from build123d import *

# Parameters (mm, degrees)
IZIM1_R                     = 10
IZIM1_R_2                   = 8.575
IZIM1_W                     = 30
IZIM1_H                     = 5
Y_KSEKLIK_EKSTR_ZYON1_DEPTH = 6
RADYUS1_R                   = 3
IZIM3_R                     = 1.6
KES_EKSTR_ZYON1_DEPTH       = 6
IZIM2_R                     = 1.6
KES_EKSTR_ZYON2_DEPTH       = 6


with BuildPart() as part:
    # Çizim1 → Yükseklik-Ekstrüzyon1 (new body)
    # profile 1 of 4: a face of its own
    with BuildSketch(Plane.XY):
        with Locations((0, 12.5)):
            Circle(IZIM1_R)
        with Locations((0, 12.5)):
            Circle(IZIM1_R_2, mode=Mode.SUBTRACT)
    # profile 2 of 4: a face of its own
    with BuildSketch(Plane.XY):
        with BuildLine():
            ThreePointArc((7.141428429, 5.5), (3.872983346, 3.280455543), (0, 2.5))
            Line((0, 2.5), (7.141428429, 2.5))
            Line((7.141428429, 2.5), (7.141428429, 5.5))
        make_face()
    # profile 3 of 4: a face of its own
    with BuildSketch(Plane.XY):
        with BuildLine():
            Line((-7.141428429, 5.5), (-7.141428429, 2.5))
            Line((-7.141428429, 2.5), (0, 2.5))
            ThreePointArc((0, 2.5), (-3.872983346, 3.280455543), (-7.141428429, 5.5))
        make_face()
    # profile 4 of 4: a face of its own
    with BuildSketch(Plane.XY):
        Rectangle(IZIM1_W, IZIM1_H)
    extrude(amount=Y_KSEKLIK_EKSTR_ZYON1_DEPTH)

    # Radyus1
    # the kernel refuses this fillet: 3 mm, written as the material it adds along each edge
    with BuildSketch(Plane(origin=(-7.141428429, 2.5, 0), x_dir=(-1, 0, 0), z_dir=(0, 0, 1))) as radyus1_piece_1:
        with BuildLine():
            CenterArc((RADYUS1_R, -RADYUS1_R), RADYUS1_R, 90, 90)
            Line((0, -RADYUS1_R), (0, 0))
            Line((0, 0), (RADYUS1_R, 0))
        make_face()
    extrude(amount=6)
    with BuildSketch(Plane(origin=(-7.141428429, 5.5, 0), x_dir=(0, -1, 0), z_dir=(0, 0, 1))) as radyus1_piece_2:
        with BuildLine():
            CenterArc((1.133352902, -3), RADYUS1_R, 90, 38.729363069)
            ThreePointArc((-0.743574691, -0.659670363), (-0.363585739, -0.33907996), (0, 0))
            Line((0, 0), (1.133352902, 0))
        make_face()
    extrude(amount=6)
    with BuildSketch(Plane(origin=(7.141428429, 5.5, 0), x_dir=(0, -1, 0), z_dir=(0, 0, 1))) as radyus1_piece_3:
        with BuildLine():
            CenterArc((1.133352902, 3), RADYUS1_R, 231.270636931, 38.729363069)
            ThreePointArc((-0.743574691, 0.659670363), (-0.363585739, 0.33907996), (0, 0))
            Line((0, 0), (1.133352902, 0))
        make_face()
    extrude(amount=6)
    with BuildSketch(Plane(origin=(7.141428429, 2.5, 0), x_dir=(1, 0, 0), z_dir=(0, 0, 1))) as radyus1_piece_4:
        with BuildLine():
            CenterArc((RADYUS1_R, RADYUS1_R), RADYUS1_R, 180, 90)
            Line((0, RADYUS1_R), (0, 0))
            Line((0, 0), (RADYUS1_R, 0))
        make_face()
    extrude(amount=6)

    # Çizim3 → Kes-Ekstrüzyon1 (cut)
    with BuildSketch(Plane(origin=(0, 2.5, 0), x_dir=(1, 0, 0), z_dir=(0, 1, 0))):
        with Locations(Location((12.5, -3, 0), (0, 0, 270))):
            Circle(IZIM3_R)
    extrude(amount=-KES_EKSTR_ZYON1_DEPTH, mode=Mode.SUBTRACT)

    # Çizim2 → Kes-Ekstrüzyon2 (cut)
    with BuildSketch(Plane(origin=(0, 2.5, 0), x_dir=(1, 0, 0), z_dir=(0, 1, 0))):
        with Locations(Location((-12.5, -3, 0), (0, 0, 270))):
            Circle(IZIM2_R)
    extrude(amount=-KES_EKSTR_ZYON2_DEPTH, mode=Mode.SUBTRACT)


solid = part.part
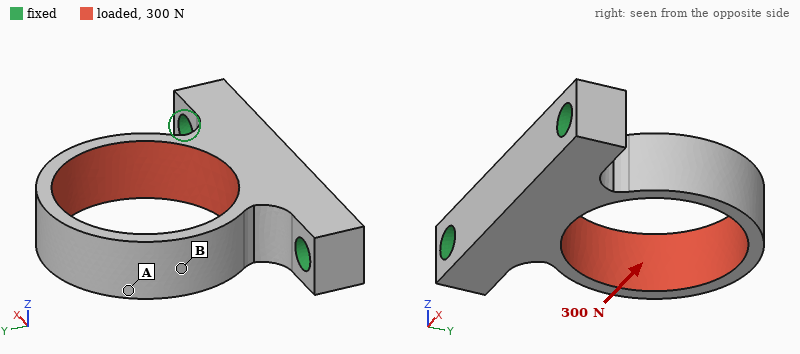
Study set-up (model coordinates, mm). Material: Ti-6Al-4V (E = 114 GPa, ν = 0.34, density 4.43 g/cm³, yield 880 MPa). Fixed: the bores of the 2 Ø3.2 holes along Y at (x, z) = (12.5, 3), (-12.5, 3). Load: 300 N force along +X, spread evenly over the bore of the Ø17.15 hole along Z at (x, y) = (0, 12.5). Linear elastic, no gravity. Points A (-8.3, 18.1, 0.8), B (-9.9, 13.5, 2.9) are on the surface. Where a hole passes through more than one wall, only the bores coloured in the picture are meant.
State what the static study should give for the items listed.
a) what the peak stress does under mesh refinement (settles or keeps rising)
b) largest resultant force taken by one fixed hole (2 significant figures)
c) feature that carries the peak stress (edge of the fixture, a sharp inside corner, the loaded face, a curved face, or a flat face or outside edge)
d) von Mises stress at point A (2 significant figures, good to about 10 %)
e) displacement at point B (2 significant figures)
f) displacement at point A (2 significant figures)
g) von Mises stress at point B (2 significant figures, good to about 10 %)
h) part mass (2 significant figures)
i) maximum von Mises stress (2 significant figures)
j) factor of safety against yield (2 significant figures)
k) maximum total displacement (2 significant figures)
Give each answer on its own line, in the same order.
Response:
settles
240 N
the loaded face
130 MPa
0.11 mm
0.15 mm
46 MPa
6.3 g
290 MPa
3.1
0.17 mm
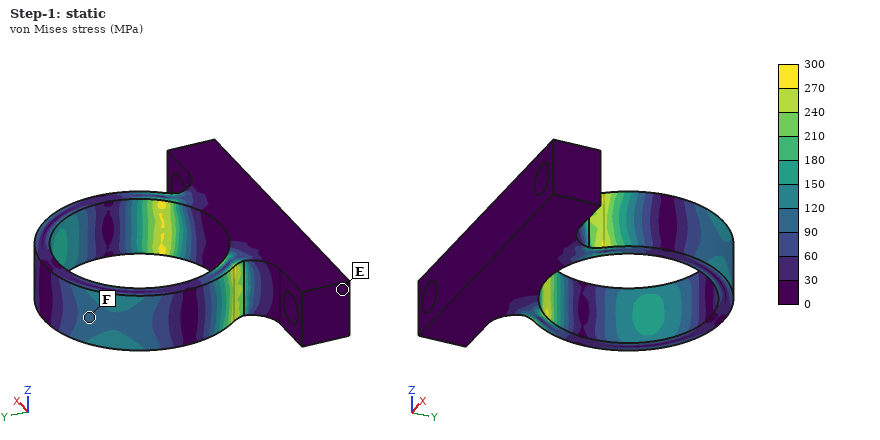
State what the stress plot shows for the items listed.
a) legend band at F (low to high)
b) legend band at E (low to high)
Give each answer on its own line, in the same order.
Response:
90 to 120 MPa
0 to 30 MPa
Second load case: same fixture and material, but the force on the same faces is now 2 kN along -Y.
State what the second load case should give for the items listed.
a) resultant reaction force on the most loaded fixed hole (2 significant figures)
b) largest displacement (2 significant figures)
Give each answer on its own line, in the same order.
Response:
1.0 kN
0.15 mm
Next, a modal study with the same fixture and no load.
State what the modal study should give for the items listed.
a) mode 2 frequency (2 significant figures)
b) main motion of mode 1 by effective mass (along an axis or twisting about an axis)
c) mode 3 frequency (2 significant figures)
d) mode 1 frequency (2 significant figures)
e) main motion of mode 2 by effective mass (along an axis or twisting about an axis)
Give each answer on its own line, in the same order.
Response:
5900 Hz
along X
13 kHz
4900 Hz
along Z
